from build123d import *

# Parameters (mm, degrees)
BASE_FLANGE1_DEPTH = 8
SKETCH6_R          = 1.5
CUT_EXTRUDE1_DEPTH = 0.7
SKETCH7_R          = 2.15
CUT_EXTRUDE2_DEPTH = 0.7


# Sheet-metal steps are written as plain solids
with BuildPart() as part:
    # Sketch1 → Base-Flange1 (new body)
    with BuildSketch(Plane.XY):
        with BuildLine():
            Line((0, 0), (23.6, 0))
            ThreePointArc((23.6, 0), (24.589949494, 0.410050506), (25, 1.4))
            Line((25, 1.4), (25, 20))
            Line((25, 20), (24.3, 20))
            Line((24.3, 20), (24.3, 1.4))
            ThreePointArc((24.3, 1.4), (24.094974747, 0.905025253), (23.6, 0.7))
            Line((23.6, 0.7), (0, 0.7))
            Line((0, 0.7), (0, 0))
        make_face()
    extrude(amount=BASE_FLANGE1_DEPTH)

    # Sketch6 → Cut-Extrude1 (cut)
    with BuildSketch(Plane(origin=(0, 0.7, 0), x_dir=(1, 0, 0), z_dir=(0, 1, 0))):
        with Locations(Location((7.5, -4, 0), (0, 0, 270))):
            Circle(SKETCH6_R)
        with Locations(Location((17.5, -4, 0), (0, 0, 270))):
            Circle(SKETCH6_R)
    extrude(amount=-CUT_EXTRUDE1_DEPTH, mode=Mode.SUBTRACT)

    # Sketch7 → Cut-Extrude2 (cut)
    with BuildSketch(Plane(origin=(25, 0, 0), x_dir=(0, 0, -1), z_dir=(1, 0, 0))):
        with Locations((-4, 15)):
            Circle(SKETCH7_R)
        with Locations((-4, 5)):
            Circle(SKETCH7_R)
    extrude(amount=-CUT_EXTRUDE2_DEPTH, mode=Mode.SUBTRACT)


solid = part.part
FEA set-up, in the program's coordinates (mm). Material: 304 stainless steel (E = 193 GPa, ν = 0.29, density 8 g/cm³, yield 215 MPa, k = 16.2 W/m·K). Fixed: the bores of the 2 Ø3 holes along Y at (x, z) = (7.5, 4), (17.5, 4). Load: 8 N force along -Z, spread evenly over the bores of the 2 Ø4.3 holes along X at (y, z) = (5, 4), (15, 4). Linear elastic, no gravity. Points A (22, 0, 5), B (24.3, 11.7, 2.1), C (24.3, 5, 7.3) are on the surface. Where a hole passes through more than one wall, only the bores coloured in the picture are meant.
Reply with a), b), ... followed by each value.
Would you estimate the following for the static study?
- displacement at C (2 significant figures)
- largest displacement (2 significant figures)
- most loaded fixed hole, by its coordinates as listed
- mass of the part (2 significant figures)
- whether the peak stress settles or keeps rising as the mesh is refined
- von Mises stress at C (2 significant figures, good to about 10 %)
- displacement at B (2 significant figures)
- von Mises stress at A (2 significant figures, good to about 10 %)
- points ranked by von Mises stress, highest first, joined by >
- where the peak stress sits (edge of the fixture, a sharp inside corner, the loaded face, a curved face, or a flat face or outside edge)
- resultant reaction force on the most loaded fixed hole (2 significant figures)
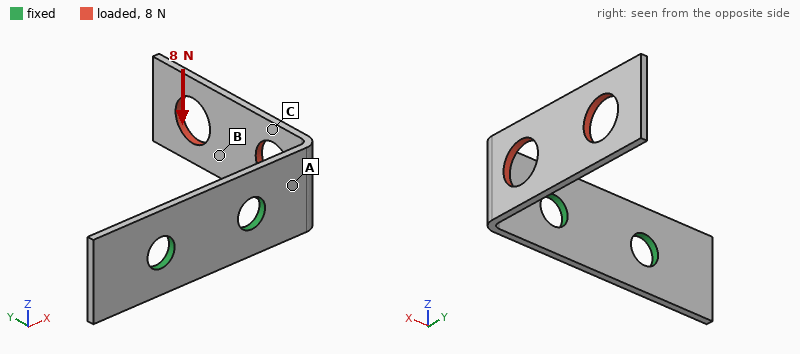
a) 0.032 mm
b) 0.11 mm
c) (17.5, 4)
d) 1.7 g
e) keeps rising
f) 22 MPa
g) 0.063 mm
h) 83 MPa
i) A > C > B
j) edge of the fixture
k) 10.0 N
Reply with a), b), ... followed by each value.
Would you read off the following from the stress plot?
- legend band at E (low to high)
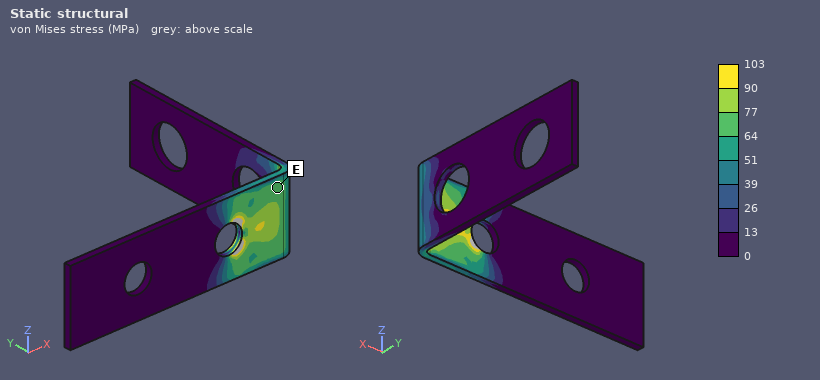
a) 64 to 77 MPa
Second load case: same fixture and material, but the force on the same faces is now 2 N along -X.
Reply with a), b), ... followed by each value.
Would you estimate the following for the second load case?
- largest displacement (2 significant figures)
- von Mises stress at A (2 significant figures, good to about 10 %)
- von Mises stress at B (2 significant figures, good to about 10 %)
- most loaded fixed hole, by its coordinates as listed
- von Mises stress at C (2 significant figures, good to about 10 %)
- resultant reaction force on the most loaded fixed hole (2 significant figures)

a) 0.10 mm
b) 26 MPa
c) 5.6 MPa
d) (17.5, 4)
e) 34 MPa
f) 1.9 N
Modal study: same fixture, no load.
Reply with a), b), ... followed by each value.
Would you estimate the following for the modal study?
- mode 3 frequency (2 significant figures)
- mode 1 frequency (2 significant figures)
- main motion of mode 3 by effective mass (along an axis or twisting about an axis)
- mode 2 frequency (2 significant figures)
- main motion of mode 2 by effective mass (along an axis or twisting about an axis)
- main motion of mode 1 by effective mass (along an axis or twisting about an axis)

a) 4900 Hz
b) 980 Hz
c) along Y
d) 1900 Hz
e) along Z
f) along X
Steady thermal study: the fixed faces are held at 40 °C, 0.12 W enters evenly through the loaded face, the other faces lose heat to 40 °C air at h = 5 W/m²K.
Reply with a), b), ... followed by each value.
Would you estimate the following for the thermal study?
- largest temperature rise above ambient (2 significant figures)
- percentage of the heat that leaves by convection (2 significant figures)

a) 21 K
b) 21 %
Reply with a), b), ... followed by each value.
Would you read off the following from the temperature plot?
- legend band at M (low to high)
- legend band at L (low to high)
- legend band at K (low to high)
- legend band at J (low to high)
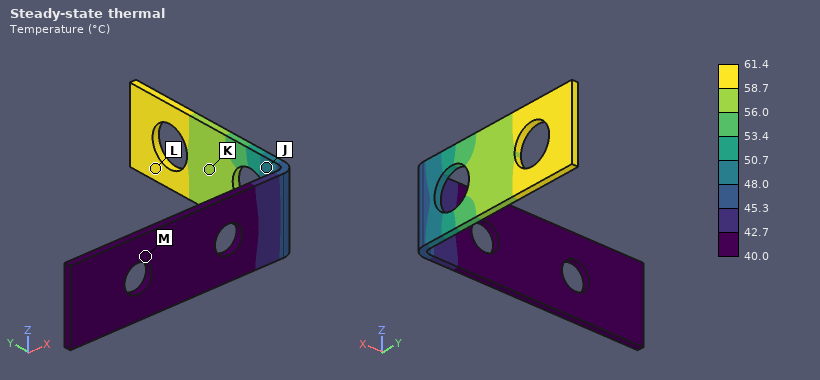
a) 40.0 to 42.7 °C
b) 58.7 to 61.4 °C
c) 56.0 to 58.7 °C
d) 48.0 to 50.7 °C
